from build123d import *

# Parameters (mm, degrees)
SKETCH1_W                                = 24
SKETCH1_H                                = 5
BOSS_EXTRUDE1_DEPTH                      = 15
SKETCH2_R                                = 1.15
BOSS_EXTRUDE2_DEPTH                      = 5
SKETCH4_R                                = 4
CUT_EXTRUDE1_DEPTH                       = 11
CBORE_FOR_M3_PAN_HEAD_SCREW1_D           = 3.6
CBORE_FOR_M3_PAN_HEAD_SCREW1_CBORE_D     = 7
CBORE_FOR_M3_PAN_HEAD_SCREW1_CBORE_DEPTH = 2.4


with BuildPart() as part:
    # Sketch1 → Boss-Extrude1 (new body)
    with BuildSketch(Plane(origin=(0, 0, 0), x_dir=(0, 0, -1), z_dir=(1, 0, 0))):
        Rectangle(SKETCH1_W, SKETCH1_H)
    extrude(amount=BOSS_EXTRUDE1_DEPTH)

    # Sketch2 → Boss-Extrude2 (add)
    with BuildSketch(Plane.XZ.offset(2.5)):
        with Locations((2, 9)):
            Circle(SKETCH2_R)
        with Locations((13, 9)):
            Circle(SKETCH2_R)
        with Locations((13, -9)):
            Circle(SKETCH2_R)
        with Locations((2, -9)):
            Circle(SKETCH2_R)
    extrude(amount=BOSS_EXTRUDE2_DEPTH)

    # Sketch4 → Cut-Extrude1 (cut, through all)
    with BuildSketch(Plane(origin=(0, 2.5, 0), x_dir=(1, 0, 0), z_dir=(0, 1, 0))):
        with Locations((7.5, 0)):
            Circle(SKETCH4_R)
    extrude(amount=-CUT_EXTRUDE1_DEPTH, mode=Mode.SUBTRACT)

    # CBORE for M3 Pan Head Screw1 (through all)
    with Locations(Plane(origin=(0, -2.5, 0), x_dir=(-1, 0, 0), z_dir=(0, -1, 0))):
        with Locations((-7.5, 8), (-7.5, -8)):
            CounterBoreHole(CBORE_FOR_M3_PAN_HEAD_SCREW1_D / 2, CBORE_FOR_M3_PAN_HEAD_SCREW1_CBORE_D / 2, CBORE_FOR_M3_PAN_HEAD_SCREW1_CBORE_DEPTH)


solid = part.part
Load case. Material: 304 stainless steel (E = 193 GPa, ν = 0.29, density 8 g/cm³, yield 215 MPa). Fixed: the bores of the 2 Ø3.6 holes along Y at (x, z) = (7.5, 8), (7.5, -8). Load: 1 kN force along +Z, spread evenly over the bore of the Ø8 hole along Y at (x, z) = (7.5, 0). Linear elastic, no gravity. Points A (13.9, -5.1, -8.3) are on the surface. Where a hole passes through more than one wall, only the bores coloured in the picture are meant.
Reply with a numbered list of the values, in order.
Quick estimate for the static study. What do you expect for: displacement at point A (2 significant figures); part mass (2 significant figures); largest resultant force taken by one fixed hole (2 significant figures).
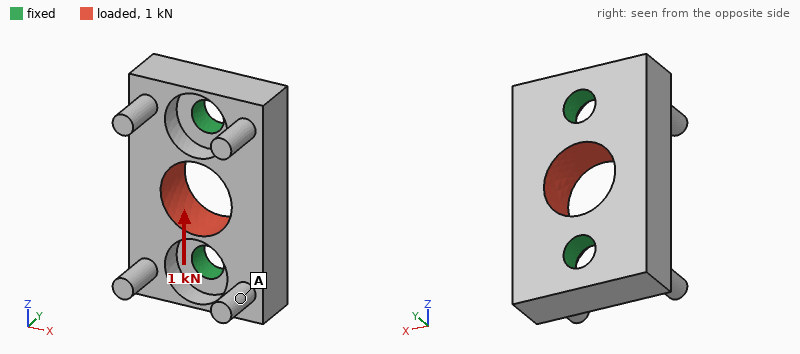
1. 0.92 µm
2. 11 g
3. 500 N
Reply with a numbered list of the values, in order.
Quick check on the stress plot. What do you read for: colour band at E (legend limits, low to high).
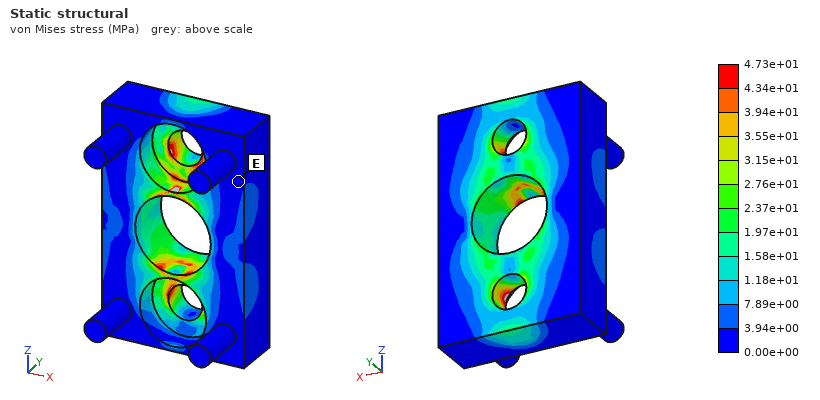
1. 0.00e+00 to 3.94e+00 MPa
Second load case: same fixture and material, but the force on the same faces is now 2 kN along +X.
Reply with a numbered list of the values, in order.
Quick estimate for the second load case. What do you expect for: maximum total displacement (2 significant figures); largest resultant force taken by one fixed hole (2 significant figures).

1. 5.7 µm
2. 1.0 kN
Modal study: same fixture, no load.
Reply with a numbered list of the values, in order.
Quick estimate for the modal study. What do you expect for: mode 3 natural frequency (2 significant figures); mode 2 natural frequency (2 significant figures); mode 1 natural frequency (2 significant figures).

1. 32 kHz
2. 31 kHz
3. 24 kHz
